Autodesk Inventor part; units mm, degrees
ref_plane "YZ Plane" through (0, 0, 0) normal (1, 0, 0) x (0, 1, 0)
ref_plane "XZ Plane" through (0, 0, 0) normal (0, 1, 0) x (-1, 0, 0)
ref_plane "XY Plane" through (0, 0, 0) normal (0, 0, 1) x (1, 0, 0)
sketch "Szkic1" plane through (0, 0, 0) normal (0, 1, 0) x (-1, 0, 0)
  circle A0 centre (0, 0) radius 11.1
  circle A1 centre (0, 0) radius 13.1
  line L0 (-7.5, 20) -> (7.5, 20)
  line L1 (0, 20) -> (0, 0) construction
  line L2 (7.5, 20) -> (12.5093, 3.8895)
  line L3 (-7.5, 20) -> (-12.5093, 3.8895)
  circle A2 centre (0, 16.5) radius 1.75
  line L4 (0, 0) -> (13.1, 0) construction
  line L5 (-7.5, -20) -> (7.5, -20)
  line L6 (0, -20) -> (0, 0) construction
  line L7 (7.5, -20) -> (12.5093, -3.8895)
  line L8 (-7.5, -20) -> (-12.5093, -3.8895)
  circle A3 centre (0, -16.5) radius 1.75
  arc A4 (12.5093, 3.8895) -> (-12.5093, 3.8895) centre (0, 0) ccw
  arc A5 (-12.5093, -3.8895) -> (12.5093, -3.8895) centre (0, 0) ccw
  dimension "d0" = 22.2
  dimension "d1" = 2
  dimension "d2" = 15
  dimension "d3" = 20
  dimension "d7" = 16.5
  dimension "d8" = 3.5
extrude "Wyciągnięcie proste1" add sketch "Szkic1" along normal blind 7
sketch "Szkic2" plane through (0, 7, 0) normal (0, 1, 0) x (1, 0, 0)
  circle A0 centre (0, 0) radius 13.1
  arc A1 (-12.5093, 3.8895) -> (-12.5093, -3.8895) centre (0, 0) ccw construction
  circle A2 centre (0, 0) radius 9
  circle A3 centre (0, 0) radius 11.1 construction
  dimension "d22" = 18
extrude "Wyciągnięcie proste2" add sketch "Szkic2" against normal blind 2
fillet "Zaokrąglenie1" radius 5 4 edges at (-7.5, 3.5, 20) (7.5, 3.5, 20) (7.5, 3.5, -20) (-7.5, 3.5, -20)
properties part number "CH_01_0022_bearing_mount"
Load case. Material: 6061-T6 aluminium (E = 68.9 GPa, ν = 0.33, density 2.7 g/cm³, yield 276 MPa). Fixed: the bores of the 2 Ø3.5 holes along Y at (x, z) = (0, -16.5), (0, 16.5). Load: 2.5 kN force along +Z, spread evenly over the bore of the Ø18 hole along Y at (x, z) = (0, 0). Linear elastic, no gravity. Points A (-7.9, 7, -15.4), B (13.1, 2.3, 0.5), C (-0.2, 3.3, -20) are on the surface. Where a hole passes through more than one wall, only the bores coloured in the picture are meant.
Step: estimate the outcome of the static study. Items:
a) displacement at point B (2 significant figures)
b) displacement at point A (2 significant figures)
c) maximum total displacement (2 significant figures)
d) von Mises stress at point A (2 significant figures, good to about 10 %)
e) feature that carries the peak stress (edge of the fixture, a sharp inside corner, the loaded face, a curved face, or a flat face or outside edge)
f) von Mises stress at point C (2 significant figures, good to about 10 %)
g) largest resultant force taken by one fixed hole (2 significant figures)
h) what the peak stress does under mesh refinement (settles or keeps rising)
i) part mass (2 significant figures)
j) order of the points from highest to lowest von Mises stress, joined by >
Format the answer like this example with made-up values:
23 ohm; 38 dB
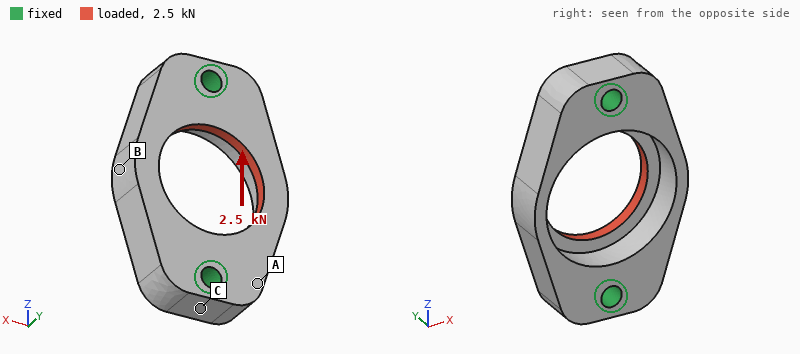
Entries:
4.4 µm; 4.3 µm; 10 µm; 13 MPa; edge of the fixture; 28 MPa; 1.3 kN; keeps rising; 8.8 g; C > A > B
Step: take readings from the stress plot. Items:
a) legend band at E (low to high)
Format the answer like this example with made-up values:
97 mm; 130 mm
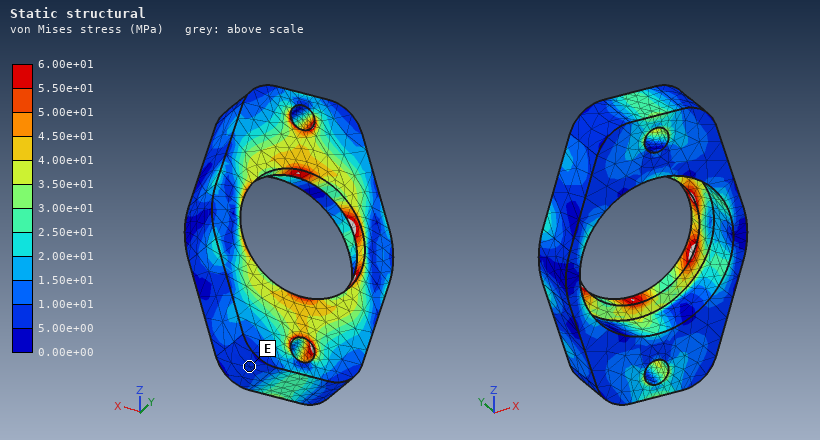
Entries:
5.00e+00 to 1.00e+01 MPa
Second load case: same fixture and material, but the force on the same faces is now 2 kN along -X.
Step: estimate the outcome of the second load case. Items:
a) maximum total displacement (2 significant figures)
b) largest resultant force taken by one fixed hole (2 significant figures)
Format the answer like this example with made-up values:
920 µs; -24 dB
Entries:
20 µm; 1.0 kN
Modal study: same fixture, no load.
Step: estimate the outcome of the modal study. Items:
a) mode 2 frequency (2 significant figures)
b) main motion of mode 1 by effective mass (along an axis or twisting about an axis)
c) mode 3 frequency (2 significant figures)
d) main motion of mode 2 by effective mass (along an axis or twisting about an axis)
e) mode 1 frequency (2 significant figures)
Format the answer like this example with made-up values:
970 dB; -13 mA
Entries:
23 kHz; twisting about Z; 28 kHz; along Y; 21 kHz
